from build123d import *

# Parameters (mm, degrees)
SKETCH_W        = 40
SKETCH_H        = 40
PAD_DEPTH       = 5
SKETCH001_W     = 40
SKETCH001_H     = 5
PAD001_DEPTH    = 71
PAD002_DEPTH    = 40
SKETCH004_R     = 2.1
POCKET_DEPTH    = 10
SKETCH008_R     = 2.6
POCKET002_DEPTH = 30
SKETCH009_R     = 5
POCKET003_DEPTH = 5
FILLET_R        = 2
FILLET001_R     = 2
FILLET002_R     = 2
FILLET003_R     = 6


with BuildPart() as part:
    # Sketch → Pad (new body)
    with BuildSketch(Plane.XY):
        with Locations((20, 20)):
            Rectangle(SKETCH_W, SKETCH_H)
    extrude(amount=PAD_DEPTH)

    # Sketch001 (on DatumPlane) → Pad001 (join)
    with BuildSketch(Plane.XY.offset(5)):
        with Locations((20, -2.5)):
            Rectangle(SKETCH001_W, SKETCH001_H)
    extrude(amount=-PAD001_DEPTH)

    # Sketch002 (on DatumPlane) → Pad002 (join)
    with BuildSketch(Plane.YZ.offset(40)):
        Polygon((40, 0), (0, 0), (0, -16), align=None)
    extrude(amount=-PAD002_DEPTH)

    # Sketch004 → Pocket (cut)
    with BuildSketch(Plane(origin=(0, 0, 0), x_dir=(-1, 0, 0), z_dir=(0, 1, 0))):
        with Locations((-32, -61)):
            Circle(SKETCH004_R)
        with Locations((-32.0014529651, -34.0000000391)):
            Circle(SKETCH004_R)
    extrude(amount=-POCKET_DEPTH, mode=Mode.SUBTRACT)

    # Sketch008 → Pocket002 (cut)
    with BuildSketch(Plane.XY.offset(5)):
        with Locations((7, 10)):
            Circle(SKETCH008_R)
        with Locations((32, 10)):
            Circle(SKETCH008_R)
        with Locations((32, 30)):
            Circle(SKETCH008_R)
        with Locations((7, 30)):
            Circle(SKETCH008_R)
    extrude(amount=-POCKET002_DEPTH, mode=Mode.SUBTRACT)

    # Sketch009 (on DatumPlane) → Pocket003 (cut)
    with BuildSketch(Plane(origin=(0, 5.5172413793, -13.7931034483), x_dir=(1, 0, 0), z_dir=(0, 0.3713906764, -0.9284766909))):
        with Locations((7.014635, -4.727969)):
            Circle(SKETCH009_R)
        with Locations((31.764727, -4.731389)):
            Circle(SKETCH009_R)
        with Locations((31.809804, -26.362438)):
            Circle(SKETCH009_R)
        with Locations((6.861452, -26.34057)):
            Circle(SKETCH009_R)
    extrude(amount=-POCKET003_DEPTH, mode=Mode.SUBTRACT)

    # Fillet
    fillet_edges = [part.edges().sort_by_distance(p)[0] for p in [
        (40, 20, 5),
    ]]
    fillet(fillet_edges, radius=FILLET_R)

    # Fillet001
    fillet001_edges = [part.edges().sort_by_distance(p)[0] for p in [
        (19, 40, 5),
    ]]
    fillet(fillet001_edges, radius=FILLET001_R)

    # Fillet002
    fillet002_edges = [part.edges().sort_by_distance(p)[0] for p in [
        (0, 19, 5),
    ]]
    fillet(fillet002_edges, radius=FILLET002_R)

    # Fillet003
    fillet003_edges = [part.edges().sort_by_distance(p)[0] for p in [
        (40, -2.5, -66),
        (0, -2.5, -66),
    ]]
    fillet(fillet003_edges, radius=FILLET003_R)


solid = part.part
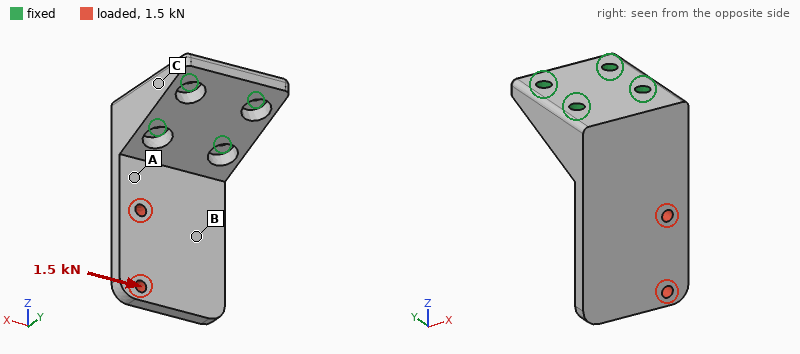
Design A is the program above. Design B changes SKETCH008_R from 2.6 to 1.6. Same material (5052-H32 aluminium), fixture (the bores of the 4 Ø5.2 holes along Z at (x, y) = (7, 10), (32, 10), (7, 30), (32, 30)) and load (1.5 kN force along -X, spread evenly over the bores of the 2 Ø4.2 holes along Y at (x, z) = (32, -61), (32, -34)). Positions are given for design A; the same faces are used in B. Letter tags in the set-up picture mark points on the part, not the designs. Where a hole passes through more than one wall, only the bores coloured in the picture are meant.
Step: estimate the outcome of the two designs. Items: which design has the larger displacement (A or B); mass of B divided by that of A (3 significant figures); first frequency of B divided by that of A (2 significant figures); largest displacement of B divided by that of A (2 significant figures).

B
1.01
1.00
1.1
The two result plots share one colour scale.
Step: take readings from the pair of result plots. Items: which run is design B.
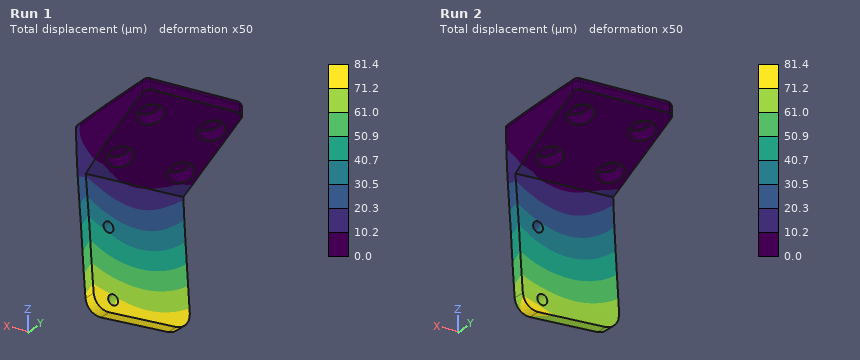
Run 1
